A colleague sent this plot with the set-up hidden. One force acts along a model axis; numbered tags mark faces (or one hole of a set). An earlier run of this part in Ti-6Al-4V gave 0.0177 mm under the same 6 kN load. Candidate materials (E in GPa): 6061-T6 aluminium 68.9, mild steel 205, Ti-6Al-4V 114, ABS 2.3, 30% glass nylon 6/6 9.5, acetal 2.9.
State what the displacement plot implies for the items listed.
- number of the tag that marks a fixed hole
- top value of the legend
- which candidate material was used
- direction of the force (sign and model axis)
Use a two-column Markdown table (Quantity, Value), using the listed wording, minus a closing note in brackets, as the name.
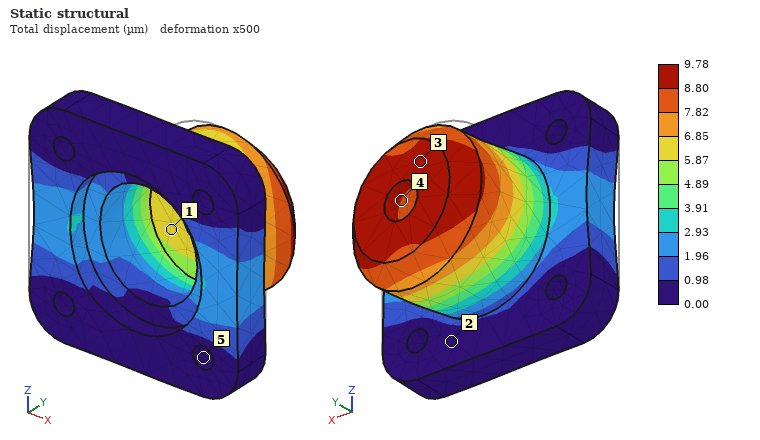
| Quantity | Value |
|---|---|
| number of the tag that marks a fixed hole | 5 |
| top value of the legend | 9.78 µm |
| which candidate material was used | mild steel |
| direction of the force | +X |
